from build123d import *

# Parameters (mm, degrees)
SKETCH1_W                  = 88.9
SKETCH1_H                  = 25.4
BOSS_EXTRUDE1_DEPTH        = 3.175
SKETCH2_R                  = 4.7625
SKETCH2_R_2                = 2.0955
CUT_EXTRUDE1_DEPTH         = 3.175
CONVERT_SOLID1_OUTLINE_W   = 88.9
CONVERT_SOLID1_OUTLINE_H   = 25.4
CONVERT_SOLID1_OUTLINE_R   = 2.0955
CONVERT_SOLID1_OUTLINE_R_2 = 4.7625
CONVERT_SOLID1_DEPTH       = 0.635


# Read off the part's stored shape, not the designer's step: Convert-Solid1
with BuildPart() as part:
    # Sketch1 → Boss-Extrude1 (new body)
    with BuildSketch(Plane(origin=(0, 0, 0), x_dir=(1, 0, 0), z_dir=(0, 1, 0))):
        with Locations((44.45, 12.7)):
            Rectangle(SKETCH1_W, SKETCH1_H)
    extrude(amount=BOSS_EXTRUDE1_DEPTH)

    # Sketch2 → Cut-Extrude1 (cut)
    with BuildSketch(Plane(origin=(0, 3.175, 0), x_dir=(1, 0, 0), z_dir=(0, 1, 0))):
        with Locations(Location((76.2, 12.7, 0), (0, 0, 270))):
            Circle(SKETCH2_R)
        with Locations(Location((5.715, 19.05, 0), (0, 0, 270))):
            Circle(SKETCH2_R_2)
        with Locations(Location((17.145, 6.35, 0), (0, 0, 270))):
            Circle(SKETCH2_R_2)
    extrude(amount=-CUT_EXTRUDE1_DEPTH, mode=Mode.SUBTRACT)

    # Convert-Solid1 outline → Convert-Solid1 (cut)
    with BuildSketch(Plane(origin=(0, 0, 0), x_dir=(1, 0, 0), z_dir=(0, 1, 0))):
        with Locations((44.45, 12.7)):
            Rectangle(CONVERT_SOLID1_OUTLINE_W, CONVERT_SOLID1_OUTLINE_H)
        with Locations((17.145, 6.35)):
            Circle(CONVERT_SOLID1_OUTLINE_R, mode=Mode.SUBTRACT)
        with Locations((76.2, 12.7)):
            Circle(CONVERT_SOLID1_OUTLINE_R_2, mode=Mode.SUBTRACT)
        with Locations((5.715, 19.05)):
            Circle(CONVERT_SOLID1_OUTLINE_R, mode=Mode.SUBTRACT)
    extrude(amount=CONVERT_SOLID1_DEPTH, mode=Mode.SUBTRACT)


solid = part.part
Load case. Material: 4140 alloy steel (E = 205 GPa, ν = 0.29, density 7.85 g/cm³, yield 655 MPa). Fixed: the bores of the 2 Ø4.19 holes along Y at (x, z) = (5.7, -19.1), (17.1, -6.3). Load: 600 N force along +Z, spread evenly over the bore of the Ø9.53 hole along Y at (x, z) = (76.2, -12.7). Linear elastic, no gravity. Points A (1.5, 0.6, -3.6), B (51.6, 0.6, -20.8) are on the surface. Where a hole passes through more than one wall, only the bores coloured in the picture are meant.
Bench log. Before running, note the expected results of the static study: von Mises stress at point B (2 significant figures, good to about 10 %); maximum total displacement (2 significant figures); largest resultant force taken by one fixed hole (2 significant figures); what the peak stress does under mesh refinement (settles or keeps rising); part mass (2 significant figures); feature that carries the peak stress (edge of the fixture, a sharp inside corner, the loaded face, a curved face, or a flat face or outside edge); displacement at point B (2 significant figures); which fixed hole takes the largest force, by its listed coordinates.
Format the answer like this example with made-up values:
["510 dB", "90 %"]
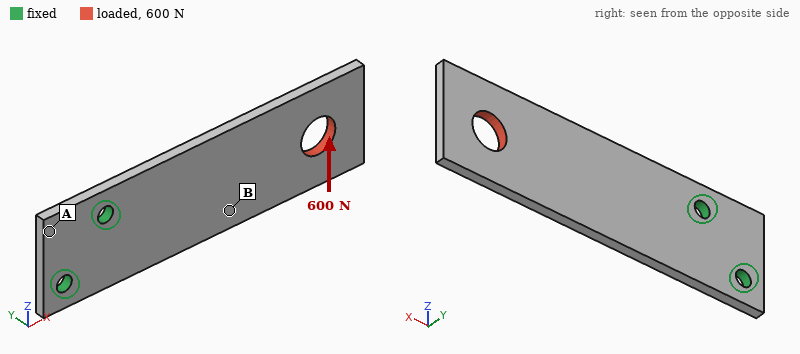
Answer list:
["37 MPa", "0.11 mm", "2.2 kN", "keeps rising", "43 g", "edge of the fixture", "0.042 mm", "(17.1, -6.3)"]
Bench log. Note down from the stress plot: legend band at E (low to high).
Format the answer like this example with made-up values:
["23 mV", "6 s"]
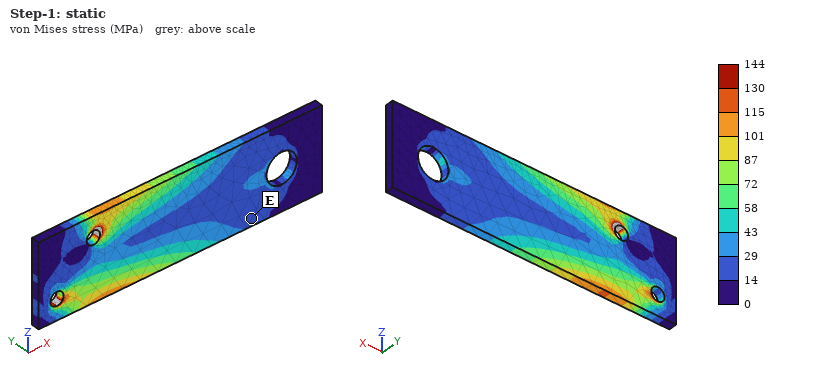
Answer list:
["14 to 29 MPa"]
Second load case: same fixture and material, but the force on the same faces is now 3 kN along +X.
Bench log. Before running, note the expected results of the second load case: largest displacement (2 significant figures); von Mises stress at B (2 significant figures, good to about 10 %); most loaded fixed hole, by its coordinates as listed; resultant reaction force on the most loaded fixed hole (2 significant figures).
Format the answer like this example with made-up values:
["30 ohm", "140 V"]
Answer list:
["21 µm", "47 MPa", "(17.1, -6.3)", "1.7 kN"]
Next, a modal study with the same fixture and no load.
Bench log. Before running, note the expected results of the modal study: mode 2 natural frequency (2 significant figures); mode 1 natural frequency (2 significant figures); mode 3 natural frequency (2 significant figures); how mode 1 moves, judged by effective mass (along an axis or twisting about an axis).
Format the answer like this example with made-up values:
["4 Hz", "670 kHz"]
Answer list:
["2100 Hz", "420 Hz", "2500 Hz", "along Y"]
